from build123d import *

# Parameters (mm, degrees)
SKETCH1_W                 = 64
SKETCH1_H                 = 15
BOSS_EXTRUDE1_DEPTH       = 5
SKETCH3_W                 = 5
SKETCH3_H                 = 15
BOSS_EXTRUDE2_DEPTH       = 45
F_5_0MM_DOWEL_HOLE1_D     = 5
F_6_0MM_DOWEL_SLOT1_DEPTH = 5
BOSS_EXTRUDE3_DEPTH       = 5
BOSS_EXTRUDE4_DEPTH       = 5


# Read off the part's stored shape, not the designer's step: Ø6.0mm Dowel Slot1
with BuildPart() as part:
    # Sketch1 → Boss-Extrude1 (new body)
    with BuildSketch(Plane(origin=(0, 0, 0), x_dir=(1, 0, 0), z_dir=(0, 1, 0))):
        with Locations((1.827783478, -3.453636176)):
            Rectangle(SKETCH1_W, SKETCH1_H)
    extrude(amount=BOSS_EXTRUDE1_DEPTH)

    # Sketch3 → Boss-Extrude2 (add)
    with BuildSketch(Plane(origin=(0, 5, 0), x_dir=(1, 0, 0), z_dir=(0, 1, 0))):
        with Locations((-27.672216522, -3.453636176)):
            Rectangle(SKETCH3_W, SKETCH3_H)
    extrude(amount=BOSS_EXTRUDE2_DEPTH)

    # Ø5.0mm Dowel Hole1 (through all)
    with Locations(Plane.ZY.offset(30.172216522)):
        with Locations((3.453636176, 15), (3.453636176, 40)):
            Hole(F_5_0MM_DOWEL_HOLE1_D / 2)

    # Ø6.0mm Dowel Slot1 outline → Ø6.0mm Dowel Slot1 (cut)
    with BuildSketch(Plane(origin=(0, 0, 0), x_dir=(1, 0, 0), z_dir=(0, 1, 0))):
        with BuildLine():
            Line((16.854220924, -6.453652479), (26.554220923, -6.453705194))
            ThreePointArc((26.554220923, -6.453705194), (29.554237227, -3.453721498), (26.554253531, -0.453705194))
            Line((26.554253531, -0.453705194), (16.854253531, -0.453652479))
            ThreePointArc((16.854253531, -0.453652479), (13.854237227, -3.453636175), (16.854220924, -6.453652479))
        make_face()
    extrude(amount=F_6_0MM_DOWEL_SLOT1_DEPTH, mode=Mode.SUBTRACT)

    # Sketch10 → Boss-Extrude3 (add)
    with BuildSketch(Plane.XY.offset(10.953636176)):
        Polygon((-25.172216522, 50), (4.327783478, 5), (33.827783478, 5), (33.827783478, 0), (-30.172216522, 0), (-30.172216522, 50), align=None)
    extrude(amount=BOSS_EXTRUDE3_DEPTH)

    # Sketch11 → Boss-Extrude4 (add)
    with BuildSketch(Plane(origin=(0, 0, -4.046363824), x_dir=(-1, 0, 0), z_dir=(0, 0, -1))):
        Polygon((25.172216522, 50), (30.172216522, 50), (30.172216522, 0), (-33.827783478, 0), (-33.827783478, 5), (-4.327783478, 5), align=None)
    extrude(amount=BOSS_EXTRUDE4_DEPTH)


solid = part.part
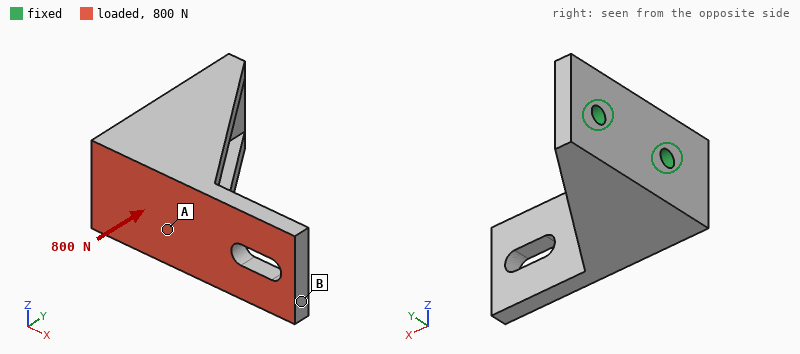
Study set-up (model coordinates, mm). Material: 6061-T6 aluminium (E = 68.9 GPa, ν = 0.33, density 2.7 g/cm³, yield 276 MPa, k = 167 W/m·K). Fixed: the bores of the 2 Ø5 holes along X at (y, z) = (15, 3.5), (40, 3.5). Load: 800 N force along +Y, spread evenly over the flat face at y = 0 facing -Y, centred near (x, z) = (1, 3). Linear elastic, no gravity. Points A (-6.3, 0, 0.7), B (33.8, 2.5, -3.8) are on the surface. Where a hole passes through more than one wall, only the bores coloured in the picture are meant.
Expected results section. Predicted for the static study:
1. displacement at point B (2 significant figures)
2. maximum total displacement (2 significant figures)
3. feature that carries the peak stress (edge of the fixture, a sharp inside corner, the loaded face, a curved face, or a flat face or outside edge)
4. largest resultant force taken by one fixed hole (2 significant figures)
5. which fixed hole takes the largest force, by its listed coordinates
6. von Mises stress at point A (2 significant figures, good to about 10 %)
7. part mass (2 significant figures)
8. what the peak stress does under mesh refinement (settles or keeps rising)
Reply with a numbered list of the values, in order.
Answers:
1. 0.17 mm
2. 0.17 mm
3. edge of the fixture
4. 940 N
5. (40, 3.5)
6. 17 MPa
7. 53 g
8. keeps rising
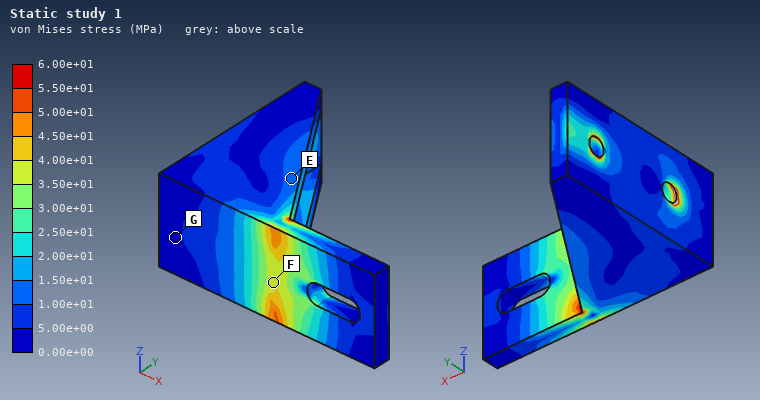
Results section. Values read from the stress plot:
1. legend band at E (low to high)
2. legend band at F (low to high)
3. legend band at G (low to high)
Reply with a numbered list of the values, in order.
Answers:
1. 1.00e+01 to 1.50e+01 MPa
2. 3.50e+01 to 4.00e+01 MPa
3. 0.00e+00 to 5.00e+00 MPa
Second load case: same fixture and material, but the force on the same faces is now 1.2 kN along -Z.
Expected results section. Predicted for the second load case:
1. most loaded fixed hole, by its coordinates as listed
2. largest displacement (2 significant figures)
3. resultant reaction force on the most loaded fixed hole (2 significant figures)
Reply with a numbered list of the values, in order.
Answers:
1. (15, 3.5)
2. 0.36 mm
3. 1.7 kN
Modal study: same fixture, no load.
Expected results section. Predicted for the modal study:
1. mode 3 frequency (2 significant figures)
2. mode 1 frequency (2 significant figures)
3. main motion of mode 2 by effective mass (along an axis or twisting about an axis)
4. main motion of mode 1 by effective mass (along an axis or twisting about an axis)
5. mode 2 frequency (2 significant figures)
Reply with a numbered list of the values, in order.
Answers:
1. 7500 Hz
2. 2300 Hz
3. along Y
4. along Z
5. 3000 Hz
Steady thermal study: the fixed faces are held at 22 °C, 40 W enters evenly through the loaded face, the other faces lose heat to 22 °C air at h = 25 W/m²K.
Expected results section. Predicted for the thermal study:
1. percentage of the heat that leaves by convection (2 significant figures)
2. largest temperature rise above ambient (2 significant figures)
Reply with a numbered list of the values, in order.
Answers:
1. 6.9 %
2. 42 K
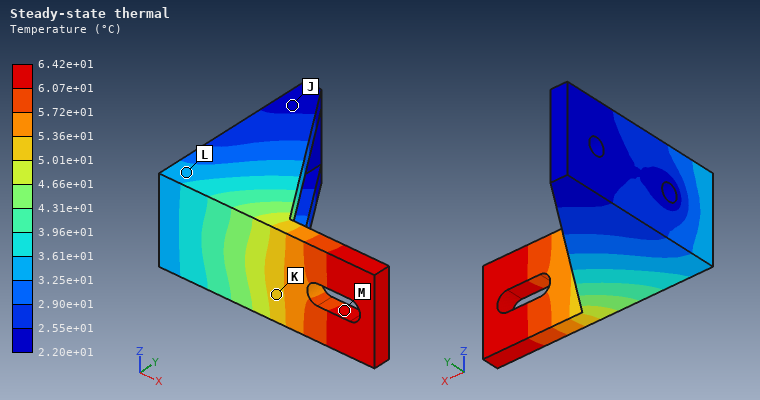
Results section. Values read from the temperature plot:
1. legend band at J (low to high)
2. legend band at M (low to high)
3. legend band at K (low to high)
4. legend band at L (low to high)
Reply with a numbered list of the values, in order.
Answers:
1. 2.20e+01 to 2.55e+01 °C
2. 6.07e+01 to 6.42e+01 °C
3. 5.01e+01 to 5.36e+01 °C
4. 3.25e+01 to 3.61e+01 °C
